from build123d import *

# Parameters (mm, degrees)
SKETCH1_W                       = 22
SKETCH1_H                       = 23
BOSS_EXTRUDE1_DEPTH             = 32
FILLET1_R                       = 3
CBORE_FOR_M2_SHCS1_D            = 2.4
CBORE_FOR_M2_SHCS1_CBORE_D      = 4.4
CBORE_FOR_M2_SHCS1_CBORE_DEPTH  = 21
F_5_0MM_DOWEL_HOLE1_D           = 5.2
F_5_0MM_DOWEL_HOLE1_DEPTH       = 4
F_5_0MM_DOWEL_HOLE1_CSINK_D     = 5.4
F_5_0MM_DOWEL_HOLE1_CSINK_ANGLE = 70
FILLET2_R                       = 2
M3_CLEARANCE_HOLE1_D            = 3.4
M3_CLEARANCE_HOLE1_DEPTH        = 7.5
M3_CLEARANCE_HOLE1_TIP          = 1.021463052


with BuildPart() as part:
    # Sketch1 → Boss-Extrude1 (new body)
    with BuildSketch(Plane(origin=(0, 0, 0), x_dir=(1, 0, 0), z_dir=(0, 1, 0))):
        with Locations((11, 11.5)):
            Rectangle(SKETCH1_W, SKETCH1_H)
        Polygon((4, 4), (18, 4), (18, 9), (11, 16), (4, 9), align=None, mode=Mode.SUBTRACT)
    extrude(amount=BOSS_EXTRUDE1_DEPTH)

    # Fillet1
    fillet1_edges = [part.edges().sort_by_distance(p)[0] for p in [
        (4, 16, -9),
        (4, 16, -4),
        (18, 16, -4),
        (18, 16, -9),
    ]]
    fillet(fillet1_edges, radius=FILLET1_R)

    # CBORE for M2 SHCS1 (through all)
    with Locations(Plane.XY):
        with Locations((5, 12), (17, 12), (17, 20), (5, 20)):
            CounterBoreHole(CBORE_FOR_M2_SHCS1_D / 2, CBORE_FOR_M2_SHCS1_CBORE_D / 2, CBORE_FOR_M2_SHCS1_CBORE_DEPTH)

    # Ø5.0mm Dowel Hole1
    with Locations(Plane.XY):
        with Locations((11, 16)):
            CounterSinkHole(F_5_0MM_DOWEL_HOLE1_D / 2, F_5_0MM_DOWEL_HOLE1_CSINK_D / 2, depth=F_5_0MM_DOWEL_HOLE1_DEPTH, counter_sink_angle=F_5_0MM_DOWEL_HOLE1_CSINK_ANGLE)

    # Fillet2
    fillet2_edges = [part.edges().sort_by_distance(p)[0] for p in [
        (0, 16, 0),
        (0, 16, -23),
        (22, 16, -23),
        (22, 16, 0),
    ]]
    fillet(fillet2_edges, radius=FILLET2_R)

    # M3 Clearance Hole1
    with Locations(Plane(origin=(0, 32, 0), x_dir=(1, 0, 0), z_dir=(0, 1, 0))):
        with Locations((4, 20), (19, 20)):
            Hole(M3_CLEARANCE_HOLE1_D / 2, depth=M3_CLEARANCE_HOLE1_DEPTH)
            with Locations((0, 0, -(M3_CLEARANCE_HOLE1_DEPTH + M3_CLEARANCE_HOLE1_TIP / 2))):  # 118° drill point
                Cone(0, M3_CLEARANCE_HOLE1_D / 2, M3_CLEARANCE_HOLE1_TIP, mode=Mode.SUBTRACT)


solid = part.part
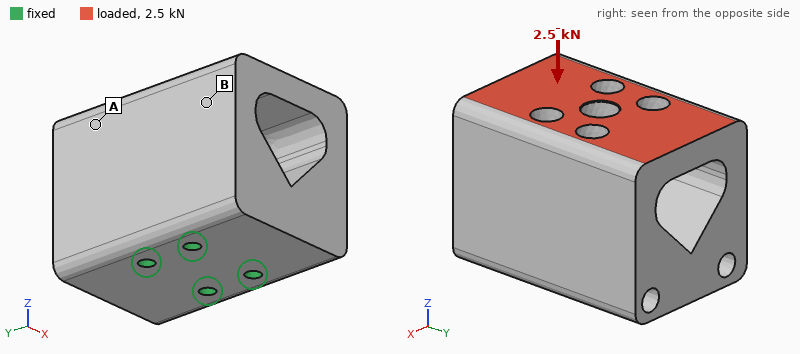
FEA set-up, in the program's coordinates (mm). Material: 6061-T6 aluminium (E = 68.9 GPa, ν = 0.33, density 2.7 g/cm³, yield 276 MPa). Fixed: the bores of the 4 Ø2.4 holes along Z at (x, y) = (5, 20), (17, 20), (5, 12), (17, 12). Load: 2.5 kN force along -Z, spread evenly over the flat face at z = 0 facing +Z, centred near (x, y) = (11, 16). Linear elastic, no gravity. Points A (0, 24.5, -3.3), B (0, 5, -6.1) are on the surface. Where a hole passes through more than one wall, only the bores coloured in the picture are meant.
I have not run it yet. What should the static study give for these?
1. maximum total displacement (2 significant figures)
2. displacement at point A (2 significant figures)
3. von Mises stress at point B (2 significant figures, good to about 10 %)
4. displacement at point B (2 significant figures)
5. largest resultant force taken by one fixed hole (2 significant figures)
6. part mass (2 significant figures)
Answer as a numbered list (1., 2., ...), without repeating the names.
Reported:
1. 15 µm
2. 5.1 µm
3. 15 MPa
4. 6.2 µm
5. 640 N
6. 30 g
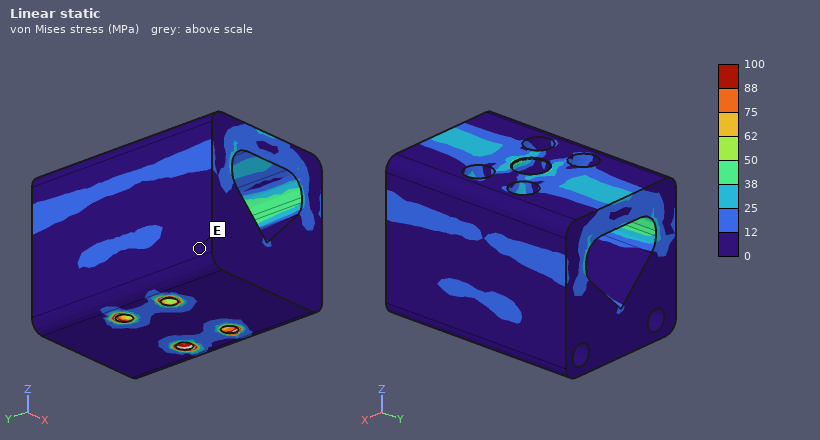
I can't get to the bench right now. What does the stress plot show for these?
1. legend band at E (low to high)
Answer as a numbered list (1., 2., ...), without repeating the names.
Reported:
1. 0 to 12 MPa
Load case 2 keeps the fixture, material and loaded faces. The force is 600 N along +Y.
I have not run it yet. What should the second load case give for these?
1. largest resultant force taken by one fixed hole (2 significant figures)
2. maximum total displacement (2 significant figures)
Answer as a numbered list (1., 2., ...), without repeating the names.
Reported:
1. 700 N
2. 30 µm
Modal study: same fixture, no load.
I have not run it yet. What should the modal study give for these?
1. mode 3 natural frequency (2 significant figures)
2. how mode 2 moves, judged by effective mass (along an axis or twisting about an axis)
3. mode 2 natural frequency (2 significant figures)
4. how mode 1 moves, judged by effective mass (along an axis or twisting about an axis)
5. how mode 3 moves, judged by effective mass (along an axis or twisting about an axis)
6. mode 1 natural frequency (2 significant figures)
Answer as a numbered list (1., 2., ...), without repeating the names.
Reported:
1. 17 kHz
2. along X
3. 9700 Hz
4. along Y
5. twisting about Z
6. 6900 Hz
